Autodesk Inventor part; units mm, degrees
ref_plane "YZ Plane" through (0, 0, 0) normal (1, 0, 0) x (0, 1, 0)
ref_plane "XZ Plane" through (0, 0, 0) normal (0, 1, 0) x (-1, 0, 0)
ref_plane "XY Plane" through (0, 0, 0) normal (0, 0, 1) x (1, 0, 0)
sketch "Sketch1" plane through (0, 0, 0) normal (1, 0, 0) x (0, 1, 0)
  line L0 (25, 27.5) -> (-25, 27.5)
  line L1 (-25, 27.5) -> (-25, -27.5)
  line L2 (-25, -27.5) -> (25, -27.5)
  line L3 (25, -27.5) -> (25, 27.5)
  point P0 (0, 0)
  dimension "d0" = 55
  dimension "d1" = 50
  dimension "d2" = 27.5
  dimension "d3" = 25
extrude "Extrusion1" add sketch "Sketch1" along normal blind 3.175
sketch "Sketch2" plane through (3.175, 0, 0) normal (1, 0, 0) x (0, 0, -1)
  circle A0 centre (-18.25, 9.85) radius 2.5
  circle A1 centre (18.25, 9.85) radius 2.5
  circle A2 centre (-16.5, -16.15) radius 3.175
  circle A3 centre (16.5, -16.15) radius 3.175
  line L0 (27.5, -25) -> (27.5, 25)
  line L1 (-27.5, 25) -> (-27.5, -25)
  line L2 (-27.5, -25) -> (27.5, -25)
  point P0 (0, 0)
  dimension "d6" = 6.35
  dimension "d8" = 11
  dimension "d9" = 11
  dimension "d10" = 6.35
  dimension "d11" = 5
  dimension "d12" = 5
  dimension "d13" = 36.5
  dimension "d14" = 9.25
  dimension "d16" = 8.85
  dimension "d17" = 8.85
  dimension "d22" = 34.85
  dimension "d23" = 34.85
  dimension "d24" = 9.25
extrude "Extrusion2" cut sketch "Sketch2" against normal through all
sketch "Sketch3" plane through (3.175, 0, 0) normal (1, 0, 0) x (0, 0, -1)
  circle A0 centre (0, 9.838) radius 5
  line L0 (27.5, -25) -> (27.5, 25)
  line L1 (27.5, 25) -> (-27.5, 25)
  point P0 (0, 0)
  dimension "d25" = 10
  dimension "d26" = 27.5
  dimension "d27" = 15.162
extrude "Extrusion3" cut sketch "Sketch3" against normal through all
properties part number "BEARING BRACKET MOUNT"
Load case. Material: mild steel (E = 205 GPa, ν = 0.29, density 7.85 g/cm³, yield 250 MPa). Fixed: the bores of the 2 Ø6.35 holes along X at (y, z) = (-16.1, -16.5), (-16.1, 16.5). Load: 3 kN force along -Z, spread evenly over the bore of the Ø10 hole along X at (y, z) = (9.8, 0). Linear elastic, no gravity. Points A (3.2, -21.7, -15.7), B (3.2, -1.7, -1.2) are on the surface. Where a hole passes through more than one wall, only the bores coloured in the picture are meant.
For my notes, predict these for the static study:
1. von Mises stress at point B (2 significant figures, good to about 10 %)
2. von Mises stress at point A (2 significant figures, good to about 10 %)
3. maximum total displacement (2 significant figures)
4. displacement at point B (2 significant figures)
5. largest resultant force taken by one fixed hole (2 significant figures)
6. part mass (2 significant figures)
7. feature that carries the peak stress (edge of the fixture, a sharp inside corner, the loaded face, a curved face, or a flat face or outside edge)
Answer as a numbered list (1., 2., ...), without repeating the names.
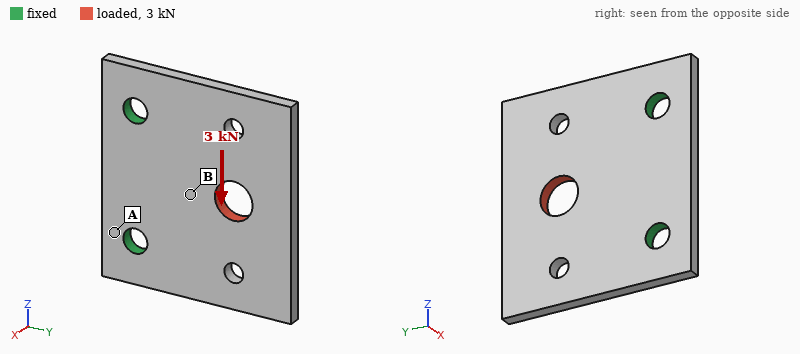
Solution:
1. 56 MPa
2. 17 MPa
3. 15 µm
4. 5.0 µm
5. 2.5 kN
6. 64 g
7. edge of the fixture
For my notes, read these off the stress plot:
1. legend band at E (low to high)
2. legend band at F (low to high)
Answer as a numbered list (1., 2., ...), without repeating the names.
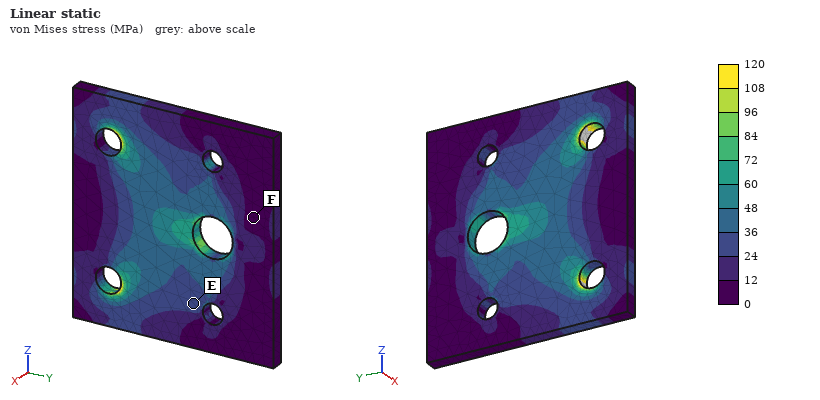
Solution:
1. 24 to 36 MPa
2. 0 to 12 MPa
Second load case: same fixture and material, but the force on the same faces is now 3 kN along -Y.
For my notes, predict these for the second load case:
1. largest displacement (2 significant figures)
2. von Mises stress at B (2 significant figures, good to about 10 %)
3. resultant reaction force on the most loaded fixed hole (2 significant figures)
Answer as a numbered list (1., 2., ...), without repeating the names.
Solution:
1. 5.8 µm
2. 25 MPa
3. 1.6 kN
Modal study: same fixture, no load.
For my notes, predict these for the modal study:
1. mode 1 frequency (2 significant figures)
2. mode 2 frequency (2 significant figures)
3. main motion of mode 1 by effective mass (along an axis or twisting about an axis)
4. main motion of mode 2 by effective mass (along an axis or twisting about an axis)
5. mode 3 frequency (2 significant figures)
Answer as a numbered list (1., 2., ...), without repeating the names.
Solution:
1. 1700 Hz
2. 3100 Hz
3. along X
4. twisting about Y
5. 7000 Hz
